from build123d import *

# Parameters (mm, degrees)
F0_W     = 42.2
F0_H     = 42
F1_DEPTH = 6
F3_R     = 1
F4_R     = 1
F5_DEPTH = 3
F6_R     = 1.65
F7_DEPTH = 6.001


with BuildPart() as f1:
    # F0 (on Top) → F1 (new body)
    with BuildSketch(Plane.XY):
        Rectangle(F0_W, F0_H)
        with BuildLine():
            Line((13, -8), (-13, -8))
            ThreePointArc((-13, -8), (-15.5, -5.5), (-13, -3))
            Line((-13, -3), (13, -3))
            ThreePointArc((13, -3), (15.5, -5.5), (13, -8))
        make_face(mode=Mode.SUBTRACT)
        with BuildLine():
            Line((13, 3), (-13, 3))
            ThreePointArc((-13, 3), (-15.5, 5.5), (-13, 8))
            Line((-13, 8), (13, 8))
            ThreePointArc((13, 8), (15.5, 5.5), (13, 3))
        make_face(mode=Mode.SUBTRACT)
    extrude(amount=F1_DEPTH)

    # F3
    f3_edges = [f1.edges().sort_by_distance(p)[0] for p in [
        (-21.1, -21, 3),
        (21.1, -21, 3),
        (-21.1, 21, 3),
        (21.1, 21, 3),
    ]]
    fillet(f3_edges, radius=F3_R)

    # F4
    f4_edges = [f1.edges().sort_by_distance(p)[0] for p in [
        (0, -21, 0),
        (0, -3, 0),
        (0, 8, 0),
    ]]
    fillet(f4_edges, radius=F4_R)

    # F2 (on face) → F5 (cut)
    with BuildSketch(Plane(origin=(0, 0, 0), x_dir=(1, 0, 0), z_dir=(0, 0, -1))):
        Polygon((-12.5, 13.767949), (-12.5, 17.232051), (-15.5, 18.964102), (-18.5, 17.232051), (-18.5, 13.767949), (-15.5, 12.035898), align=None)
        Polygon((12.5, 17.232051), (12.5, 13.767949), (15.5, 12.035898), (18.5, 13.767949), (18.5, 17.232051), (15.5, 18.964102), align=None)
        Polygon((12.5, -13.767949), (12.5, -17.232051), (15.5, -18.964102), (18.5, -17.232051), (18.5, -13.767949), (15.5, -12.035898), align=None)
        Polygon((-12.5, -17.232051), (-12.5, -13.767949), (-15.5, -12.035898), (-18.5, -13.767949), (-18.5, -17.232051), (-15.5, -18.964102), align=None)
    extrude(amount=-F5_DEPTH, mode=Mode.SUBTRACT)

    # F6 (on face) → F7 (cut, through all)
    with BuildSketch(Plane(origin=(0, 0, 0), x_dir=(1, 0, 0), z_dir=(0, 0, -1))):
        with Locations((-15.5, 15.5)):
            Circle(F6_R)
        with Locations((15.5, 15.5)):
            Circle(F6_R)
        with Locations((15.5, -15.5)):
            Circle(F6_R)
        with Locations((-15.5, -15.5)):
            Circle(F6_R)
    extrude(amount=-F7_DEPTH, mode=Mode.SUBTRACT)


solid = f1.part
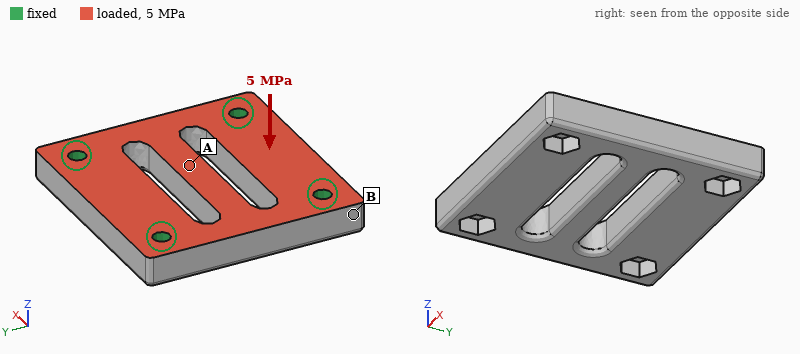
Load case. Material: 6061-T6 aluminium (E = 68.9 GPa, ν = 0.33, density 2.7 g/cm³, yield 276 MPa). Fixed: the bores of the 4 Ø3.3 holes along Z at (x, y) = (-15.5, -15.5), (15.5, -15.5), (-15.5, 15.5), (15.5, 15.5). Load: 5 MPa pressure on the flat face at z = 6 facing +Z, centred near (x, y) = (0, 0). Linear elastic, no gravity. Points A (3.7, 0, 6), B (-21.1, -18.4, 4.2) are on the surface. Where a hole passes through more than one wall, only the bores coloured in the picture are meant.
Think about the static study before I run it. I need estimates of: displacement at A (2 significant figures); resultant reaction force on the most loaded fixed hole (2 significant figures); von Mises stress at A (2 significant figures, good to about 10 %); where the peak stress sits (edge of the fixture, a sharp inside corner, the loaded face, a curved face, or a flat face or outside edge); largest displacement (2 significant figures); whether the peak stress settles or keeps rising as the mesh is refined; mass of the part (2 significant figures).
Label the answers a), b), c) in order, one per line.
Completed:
a) 74 µm
b) 1.9 kN
c) 72 MPa
d) edge of the fixture
e) 78 µm
f) keeps rising
g) 22 g
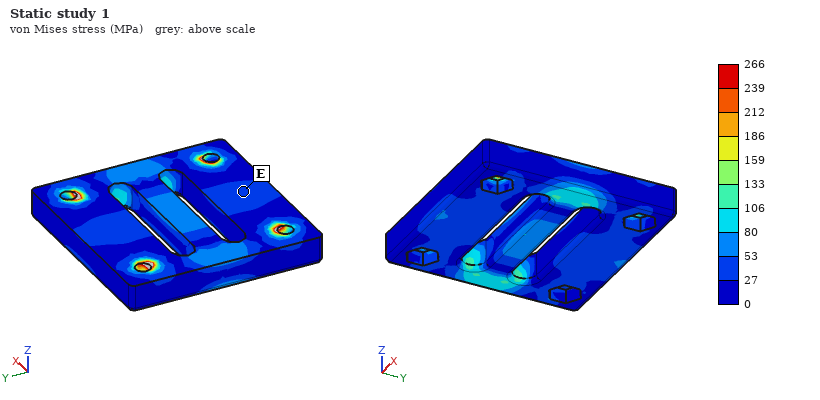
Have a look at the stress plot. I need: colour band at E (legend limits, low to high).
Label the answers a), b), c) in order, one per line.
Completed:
a) 27 to 53 MPa
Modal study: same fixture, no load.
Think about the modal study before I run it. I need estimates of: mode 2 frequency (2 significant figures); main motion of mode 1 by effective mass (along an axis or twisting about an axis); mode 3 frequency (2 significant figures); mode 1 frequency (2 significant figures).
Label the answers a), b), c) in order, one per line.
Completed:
a) 20 kHz
b) along Z
c) 21 kHz
d) 12 kHz
